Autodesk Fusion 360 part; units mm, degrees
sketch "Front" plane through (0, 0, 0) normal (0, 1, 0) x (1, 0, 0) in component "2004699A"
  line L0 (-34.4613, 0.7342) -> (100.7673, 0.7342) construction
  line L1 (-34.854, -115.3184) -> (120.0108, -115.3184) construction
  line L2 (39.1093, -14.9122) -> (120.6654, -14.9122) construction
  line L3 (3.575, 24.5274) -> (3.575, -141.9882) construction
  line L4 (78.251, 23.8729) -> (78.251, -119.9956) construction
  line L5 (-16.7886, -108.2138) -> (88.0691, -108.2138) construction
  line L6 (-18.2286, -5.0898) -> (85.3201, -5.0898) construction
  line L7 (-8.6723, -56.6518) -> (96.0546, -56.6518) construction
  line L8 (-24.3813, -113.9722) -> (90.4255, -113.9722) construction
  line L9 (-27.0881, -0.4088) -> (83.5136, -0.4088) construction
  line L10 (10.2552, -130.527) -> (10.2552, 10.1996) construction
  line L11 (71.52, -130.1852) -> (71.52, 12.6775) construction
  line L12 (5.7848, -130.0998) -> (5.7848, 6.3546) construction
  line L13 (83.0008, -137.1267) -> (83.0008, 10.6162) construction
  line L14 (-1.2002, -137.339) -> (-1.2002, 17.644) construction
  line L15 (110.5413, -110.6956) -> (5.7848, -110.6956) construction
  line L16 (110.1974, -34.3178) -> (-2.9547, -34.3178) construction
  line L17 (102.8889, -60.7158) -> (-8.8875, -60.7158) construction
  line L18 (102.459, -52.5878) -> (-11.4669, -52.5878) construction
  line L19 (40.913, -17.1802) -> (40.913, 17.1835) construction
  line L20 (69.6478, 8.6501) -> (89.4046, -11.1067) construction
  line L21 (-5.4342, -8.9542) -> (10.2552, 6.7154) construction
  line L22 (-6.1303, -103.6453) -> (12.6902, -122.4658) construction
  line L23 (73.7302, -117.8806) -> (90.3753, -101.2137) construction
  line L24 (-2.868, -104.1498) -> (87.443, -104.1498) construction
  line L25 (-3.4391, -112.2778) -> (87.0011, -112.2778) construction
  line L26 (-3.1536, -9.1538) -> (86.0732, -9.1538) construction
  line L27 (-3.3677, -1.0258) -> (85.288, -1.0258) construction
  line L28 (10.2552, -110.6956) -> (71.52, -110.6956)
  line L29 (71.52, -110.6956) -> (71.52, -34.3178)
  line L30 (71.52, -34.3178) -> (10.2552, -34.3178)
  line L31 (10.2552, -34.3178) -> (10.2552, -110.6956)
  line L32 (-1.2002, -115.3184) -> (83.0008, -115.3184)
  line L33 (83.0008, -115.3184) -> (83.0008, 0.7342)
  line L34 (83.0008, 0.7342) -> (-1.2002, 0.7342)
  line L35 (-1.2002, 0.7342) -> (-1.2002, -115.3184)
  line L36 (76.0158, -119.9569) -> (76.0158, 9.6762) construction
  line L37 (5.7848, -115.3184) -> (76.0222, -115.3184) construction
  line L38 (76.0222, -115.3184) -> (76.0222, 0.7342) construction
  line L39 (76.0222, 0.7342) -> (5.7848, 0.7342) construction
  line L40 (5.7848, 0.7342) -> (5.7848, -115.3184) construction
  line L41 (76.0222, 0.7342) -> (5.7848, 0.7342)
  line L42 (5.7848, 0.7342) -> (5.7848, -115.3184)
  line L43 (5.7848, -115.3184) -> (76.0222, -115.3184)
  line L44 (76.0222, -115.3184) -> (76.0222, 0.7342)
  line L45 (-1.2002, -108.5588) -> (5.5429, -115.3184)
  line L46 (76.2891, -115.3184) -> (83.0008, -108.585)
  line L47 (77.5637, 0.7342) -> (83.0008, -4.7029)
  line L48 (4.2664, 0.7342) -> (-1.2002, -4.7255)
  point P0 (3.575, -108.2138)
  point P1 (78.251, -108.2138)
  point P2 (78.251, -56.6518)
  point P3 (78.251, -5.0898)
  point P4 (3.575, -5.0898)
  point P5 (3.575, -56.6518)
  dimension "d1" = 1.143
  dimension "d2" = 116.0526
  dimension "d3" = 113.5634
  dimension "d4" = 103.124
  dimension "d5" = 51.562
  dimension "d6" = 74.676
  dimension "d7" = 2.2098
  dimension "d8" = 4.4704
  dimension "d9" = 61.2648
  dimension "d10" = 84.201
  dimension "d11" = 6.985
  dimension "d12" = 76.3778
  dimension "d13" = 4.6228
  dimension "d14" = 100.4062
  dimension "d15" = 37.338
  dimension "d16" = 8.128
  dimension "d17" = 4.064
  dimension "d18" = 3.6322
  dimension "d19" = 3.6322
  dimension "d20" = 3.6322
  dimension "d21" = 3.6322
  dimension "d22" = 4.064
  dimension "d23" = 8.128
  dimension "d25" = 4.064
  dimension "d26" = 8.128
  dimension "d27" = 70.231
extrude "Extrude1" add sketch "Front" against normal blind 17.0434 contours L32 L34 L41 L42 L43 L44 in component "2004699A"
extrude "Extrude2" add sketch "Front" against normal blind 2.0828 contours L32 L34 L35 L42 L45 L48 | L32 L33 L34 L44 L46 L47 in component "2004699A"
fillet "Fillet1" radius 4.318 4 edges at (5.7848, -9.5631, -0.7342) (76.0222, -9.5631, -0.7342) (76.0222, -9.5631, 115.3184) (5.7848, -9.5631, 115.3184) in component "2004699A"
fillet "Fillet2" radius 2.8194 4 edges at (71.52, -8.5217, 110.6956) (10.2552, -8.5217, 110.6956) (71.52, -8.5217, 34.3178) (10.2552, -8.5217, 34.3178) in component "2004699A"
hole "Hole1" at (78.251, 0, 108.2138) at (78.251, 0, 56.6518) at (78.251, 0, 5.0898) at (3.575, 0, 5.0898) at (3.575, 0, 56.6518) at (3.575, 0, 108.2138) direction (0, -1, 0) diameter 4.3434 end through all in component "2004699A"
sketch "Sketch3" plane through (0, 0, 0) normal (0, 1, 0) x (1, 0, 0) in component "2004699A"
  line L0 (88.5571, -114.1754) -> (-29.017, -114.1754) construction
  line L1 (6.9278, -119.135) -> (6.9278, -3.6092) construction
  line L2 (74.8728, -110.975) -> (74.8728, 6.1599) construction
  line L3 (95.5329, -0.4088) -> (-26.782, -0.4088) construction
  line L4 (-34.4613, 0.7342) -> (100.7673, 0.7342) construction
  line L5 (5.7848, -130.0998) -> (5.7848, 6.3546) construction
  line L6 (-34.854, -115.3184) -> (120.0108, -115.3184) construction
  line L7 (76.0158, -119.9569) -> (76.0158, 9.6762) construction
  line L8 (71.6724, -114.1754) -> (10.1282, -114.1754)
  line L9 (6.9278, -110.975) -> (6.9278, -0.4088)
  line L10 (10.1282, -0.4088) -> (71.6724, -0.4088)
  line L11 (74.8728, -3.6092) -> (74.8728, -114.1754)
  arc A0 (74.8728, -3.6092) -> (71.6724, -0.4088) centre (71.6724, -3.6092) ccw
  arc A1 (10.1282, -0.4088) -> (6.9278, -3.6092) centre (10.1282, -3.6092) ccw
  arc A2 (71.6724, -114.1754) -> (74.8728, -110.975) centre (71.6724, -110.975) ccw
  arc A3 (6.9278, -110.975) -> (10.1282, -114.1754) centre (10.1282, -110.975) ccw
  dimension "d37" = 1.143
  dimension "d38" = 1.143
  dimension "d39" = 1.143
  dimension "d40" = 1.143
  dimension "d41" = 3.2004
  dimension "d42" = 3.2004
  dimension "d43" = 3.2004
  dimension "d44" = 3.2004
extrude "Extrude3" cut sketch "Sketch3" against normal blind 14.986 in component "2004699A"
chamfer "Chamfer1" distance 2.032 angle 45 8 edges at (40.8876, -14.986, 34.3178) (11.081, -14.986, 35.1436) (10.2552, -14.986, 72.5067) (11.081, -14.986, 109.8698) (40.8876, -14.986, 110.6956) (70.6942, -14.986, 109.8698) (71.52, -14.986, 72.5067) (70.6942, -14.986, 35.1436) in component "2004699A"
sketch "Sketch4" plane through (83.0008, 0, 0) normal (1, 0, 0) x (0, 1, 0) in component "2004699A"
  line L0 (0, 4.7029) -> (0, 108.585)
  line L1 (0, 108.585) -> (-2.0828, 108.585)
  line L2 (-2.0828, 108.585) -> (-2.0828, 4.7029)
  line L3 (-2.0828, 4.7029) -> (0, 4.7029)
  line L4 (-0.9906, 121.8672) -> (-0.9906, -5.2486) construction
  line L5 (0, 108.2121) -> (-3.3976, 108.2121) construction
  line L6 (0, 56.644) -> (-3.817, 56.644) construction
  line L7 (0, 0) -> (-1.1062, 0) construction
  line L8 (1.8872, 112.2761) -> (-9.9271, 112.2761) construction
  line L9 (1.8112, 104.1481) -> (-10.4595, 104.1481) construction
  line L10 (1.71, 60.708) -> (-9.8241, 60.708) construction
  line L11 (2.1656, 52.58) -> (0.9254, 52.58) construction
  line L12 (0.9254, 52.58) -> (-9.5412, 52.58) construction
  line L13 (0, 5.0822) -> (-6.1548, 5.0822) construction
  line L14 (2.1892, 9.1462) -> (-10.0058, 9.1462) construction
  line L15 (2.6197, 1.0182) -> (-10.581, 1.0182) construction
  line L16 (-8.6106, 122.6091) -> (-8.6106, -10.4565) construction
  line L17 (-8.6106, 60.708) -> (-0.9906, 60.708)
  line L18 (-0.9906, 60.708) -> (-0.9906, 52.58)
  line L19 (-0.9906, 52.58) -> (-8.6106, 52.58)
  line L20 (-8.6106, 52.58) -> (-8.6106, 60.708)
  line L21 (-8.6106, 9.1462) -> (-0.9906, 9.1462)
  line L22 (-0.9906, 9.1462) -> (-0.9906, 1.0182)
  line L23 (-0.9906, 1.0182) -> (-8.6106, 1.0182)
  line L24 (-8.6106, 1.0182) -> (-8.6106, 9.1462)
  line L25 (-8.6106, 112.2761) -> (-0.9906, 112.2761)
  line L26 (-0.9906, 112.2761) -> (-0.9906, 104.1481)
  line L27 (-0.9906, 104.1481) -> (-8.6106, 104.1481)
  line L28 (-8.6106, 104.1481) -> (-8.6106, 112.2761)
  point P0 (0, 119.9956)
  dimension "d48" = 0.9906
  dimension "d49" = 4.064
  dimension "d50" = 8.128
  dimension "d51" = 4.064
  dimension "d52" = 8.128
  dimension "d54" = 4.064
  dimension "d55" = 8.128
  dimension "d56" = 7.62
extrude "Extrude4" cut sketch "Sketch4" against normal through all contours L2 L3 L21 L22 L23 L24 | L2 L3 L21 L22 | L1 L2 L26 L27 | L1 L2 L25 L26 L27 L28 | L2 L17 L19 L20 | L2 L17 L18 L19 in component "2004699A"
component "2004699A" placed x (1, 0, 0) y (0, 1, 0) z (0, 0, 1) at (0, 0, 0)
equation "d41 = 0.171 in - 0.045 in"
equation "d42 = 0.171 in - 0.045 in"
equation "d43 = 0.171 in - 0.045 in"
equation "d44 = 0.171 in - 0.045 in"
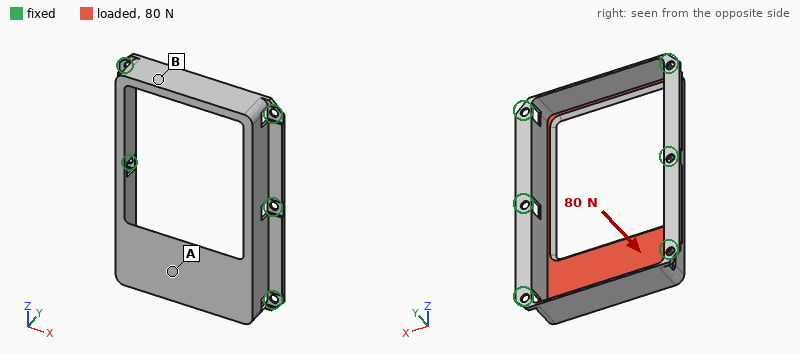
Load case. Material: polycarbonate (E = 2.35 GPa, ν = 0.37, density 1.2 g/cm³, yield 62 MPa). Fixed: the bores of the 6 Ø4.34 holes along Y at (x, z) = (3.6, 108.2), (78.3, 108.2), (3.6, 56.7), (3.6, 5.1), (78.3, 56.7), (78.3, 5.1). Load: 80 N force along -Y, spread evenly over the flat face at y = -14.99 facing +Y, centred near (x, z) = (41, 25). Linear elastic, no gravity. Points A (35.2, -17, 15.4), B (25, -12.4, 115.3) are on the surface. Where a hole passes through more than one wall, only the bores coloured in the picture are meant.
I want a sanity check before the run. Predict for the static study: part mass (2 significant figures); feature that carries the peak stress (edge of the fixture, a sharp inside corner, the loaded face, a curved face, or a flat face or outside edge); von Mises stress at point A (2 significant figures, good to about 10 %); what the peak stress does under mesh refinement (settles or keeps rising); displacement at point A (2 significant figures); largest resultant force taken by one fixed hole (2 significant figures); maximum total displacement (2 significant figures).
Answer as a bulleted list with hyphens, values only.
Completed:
- 18 g
- edge of the fixture
- 5.6 MPa
- keeps rising
- 0.85 mm
- 33 N
- 1.7 mm
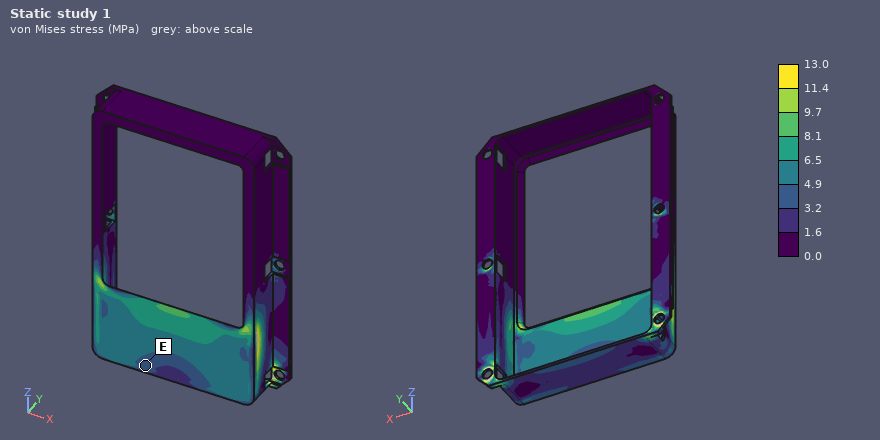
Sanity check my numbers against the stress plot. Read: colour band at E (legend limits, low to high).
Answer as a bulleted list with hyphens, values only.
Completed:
- 3.2 to 4.9 MPa
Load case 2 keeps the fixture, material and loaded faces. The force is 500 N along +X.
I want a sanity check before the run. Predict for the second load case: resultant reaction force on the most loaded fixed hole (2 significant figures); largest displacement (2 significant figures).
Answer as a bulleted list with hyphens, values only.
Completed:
- 250 N
- 1.1 mm
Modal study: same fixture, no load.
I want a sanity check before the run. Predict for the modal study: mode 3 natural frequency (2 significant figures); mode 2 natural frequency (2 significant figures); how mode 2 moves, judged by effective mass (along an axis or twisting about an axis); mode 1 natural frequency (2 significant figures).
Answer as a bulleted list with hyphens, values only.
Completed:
- 880 Hz
- 580 Hz
- along Y
- 540 Hz
